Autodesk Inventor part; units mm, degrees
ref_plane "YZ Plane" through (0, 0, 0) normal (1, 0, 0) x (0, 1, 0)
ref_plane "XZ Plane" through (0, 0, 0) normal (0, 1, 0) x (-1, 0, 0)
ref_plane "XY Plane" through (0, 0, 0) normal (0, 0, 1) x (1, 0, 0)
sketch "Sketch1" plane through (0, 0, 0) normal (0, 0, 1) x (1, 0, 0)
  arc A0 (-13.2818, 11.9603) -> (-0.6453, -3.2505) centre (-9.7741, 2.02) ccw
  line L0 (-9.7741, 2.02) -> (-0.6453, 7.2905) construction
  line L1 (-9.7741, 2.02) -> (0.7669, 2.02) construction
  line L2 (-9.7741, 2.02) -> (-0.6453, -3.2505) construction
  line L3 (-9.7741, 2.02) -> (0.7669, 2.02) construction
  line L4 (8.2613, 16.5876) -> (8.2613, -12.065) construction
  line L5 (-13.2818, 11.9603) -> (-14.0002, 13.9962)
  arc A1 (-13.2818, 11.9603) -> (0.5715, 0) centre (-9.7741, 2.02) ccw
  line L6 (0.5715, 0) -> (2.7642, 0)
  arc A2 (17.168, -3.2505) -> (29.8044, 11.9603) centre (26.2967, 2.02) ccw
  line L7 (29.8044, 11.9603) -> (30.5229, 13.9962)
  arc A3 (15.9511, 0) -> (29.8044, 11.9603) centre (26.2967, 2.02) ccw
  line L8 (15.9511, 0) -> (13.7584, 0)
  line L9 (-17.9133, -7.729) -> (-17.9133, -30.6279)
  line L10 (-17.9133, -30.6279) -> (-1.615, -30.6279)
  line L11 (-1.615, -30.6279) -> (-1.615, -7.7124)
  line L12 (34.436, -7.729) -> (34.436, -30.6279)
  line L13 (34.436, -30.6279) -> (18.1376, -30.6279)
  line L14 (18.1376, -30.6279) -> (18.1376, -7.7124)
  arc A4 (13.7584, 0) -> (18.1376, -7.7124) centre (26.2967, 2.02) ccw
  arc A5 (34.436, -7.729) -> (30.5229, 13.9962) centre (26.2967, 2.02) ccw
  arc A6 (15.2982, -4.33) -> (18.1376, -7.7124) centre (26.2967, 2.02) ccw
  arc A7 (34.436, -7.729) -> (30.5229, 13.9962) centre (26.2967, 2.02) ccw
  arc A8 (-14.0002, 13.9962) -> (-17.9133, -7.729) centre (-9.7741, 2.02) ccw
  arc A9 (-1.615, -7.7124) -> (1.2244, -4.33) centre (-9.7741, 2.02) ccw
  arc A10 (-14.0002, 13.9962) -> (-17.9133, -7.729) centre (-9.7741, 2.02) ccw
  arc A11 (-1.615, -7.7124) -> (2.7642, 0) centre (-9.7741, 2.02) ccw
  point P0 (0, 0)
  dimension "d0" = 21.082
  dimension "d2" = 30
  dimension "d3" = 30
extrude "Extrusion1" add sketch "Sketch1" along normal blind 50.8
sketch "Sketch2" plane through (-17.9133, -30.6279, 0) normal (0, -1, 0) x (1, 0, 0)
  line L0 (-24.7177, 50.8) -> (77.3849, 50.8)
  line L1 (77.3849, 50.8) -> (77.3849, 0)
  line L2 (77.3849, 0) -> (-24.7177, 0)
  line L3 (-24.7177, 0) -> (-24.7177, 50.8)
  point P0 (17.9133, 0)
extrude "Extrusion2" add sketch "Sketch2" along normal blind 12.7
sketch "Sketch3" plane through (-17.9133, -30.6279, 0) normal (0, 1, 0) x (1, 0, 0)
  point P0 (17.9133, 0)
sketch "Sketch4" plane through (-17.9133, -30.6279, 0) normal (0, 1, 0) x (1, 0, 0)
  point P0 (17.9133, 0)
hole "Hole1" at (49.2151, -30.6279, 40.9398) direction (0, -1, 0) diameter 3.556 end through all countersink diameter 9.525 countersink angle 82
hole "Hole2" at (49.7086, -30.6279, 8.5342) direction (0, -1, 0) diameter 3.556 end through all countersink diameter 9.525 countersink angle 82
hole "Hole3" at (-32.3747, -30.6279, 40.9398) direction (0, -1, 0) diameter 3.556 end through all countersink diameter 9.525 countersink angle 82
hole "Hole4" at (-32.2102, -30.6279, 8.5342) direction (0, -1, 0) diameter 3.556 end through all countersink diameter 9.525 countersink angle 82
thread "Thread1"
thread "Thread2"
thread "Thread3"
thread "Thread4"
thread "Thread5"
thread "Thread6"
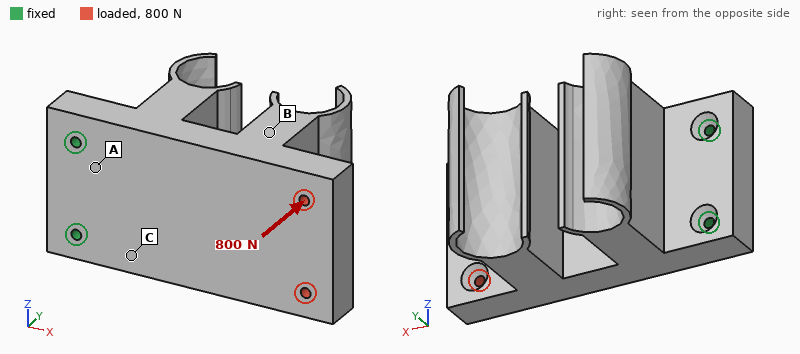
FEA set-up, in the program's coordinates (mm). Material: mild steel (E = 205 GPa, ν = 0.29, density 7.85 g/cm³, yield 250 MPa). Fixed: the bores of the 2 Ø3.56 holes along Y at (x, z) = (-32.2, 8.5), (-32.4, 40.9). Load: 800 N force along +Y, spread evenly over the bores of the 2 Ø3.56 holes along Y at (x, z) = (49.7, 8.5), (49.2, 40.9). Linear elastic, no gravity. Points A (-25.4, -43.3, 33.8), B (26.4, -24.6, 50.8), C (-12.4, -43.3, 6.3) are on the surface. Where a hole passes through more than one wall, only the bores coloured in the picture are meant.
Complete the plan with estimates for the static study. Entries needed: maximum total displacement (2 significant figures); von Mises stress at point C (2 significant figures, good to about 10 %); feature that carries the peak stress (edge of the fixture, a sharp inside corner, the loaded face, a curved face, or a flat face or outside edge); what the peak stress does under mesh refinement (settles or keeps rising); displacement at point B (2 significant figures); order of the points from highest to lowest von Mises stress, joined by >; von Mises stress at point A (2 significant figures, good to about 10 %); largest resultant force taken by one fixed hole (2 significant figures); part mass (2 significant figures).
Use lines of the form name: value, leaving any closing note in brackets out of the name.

maximum total displacement: 0.12 mm
von Mises stress at point C: 25 MPa
feature that carries the peak stress: edge of the fixture
what the peak stress does under mesh refinement: keeps rising
displacement at point B: 0.070 mm
order of the points from highest to lowest von Mises stress, joined by >: A > C > B
von Mises stress at point A: 37 MPa
largest resultant force taken by one fixed hole: 410 N
part mass: 870 g
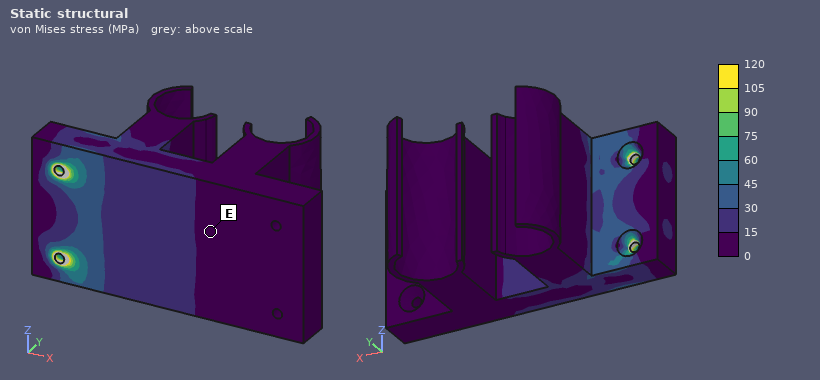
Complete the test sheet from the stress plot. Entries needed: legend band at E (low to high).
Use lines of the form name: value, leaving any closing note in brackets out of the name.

legend band at E: 0 to 15 MPa
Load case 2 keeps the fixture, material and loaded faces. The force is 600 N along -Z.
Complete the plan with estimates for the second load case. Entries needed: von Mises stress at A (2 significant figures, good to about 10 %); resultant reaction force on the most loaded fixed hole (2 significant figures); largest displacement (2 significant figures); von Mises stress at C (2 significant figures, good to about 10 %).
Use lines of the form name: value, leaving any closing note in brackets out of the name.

von Mises stress at A: 5.8 MPa
resultant reaction force on the most loaded fixed hole: 1.5 kN
largest displacement: 7.6 µm
von Mises stress at C: 6.2 MPa
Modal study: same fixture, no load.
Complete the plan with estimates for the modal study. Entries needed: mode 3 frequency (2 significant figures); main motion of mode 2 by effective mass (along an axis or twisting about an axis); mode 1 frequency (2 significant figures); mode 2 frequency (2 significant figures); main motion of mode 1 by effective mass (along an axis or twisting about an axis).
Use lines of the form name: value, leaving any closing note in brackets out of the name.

mode 3 frequency: 2900 Hz
main motion of mode 2 by effective mass: along Z
mode 1 frequency: 820 Hz
mode 2 frequency: 2700 Hz
main motion of mode 1 by effective mass: along Y
